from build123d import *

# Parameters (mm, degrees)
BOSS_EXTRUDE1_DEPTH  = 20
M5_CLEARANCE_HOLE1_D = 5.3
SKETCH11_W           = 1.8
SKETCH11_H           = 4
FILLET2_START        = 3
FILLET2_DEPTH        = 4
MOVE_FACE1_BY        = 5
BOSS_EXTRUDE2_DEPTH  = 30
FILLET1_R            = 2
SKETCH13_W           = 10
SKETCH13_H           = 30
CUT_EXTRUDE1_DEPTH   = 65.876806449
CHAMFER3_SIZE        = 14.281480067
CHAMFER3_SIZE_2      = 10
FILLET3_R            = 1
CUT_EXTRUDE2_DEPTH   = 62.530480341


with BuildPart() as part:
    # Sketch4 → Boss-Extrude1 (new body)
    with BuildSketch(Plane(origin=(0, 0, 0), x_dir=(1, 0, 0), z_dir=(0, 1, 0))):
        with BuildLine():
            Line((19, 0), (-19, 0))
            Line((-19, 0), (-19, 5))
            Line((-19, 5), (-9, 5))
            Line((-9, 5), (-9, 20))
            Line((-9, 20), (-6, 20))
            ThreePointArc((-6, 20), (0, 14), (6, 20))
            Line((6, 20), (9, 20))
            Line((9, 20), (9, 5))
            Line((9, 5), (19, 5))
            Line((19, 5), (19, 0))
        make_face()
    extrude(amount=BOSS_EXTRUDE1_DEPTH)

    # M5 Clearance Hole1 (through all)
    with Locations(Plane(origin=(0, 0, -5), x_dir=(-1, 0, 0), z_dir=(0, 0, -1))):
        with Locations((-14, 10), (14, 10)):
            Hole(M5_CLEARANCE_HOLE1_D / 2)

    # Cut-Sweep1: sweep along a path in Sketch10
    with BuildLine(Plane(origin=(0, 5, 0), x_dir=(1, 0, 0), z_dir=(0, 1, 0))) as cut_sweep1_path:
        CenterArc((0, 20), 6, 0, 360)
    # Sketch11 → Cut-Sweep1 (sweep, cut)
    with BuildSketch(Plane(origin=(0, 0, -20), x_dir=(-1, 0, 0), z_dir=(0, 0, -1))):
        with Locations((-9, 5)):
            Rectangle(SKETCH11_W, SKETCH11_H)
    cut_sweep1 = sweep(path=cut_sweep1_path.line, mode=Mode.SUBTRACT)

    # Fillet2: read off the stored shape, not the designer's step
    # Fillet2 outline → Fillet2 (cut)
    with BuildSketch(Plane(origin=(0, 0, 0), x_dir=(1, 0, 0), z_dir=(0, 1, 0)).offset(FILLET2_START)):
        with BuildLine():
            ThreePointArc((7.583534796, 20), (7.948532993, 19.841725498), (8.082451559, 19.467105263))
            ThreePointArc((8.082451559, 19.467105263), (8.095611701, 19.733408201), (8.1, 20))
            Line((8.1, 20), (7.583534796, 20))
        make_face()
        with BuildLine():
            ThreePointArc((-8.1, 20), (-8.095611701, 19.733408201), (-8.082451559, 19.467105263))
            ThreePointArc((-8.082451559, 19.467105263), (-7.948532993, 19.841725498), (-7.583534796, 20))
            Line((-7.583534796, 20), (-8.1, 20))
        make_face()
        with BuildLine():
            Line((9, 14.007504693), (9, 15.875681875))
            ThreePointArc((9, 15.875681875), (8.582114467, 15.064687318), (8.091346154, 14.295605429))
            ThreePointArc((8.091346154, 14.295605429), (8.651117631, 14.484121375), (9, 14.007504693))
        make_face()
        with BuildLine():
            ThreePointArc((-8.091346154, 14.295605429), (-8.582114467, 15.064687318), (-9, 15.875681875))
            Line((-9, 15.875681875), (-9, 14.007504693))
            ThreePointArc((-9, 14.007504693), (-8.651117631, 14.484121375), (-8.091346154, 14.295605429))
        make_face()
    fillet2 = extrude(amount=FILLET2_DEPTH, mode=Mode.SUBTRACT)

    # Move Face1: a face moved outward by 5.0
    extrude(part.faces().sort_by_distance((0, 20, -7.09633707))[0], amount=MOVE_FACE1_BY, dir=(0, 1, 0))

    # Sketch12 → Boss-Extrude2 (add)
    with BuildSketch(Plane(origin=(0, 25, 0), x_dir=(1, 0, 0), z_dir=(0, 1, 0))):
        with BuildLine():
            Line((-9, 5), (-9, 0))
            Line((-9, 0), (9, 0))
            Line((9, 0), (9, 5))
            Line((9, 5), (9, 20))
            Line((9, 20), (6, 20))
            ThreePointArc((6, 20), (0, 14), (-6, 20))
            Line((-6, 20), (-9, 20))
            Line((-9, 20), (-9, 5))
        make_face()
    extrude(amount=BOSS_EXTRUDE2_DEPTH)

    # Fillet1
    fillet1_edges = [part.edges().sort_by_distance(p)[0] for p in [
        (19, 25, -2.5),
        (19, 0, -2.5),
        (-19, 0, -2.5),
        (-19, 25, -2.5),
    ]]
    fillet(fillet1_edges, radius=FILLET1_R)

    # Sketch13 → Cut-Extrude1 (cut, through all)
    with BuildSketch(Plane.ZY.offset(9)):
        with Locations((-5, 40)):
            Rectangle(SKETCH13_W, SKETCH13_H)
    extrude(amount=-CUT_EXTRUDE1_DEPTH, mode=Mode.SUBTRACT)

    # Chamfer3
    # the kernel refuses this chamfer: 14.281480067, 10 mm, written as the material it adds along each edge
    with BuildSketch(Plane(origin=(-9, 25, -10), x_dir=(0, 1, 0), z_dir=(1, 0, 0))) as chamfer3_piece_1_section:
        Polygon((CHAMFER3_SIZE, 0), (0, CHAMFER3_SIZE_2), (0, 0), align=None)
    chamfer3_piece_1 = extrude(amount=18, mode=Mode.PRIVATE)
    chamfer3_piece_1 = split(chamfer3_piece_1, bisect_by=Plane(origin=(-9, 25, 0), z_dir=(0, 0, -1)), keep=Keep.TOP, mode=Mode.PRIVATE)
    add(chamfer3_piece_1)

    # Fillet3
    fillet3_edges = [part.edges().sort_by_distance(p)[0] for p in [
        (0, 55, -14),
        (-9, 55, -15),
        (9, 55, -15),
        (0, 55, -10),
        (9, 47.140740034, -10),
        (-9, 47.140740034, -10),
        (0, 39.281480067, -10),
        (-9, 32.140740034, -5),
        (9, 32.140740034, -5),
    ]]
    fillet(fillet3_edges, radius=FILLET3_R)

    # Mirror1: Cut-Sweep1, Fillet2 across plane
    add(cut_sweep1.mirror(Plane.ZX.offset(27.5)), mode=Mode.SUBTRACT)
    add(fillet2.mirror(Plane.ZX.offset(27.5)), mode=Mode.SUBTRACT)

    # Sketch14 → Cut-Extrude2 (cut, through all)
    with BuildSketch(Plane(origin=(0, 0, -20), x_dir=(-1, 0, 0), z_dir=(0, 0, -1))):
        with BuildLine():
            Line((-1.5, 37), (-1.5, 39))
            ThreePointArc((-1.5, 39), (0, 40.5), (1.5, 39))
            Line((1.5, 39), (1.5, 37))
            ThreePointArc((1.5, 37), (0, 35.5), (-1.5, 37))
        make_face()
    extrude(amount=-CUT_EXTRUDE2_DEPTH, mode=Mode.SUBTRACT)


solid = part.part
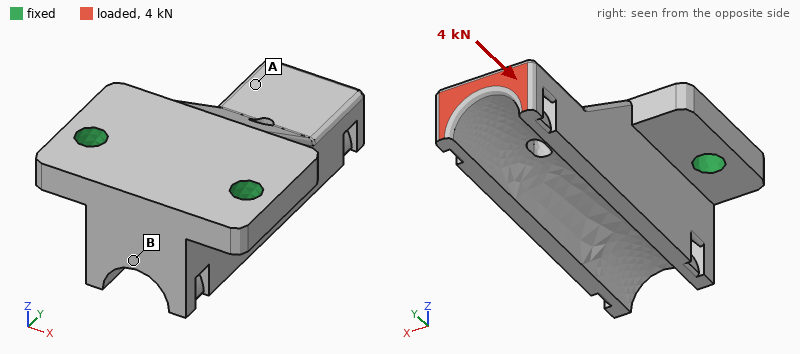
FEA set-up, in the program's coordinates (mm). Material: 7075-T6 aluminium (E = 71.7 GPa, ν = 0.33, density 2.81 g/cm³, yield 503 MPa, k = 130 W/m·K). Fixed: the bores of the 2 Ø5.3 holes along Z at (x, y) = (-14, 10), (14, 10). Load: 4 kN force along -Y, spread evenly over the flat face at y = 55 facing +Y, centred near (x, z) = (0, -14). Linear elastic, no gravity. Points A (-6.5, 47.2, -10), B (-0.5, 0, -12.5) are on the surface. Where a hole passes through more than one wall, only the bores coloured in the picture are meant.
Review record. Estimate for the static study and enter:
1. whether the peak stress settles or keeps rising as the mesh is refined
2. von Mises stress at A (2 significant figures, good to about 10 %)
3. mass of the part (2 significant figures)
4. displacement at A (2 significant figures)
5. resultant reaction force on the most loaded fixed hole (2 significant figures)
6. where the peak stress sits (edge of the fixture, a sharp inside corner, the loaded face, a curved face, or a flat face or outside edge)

keeps rising
53 MPa
40 g
0.21 mm
2.0 kN
edge of the fixture
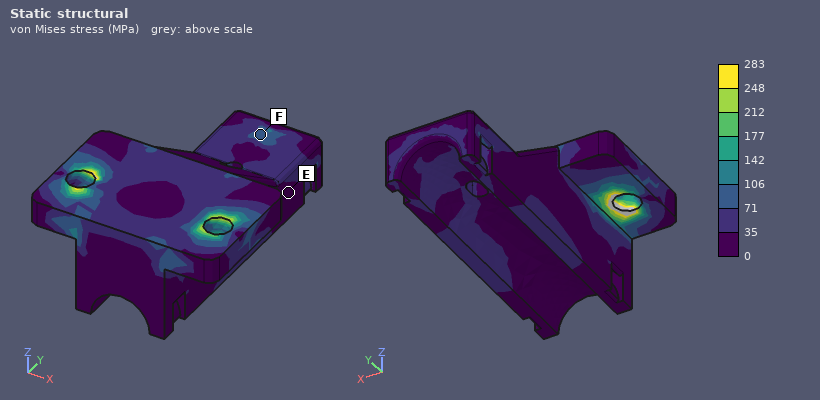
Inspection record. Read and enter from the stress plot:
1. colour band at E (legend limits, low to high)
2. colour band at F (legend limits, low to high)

0 to 35 MPa
71 to 106 MPa
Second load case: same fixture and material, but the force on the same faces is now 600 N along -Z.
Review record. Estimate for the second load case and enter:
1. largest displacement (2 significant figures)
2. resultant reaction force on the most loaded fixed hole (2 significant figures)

0.21 mm
380 N
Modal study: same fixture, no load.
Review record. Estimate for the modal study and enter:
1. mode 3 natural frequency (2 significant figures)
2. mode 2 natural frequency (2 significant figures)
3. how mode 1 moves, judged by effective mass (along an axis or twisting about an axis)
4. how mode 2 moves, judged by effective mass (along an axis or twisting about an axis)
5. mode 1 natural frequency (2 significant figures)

16 kHz
9200 Hz
along Z
along X
3800 Hz
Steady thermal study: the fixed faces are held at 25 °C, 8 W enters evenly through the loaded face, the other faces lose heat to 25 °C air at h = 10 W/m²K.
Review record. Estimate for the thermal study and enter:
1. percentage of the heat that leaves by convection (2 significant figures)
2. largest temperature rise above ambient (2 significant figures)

4.0 %
19 K
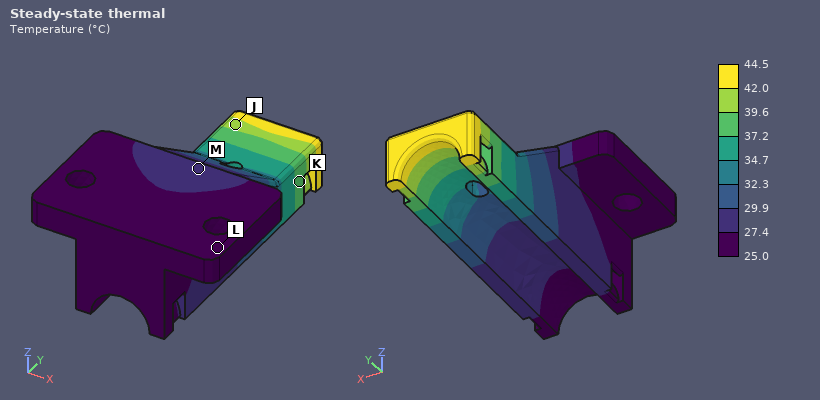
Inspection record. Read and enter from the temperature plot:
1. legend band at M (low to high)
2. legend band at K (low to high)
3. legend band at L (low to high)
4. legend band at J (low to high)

27.4 to 29.9 °C
37.2 to 39.6 °C
25.0 to 27.4 °C
39.6 to 42.0 °C
